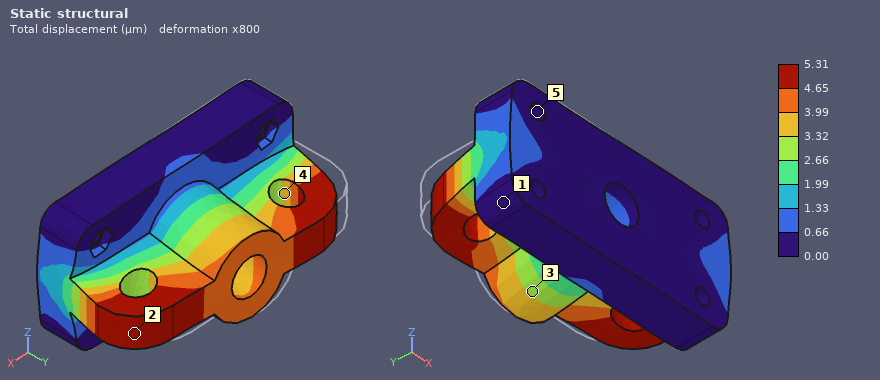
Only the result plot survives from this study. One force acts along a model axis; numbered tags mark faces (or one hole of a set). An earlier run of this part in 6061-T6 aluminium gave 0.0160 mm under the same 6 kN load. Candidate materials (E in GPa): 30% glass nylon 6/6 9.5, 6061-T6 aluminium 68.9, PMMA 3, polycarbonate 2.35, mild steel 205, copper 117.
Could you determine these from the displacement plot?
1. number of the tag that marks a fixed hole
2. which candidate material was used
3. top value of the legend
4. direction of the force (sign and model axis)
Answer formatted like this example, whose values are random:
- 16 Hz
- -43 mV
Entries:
- 5
- mild steel
- 5.31 µm
- +X
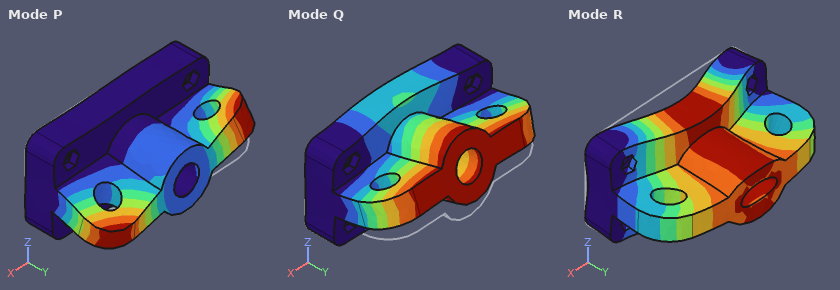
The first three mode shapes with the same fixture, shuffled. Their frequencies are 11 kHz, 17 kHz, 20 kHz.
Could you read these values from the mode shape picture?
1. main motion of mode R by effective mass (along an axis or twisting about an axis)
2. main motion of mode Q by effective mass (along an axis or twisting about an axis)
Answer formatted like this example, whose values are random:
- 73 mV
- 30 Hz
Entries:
- along Y
- along Z
